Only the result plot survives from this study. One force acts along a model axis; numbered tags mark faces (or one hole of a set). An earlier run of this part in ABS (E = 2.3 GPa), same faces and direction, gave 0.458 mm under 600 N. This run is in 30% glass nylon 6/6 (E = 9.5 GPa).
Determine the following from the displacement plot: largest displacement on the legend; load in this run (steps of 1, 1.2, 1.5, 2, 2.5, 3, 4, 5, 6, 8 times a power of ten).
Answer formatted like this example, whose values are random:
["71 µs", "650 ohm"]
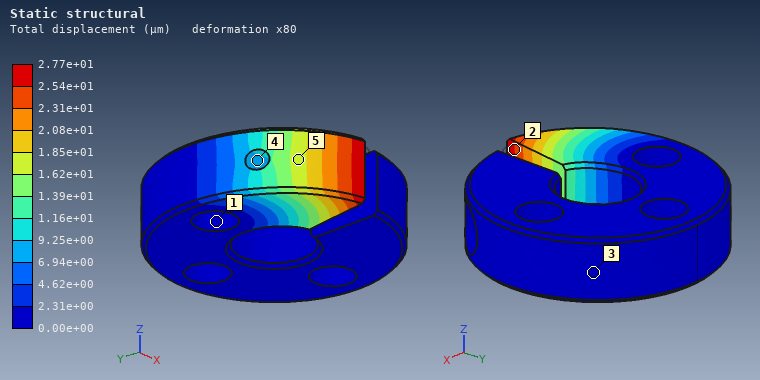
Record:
["2.77e+01 µm", "150 N"]
